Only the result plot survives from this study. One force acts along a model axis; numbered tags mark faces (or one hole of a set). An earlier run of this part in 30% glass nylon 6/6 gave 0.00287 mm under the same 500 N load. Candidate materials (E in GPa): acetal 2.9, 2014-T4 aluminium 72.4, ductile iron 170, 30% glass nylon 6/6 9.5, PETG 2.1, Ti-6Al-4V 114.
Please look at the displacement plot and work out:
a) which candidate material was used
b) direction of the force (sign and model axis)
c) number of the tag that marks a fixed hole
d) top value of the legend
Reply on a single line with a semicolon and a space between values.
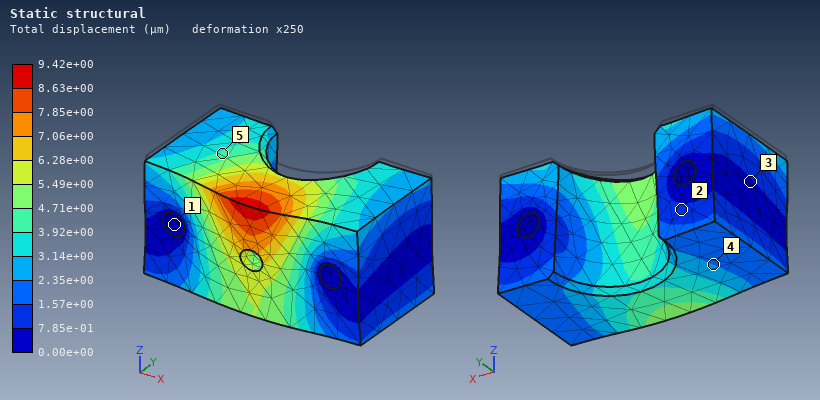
acetal; -Z; 1; 9.42e+00 µm
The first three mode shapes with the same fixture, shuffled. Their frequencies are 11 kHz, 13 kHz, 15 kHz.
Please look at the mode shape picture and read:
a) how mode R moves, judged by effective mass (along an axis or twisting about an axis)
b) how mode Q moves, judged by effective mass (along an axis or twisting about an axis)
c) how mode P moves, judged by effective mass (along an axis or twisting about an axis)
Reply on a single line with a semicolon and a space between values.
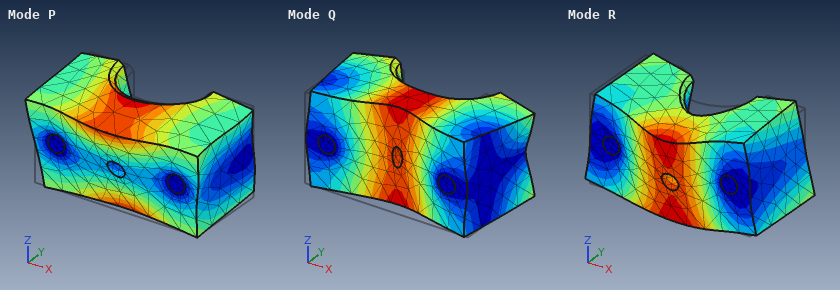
along Z; along Y; twisting about X
